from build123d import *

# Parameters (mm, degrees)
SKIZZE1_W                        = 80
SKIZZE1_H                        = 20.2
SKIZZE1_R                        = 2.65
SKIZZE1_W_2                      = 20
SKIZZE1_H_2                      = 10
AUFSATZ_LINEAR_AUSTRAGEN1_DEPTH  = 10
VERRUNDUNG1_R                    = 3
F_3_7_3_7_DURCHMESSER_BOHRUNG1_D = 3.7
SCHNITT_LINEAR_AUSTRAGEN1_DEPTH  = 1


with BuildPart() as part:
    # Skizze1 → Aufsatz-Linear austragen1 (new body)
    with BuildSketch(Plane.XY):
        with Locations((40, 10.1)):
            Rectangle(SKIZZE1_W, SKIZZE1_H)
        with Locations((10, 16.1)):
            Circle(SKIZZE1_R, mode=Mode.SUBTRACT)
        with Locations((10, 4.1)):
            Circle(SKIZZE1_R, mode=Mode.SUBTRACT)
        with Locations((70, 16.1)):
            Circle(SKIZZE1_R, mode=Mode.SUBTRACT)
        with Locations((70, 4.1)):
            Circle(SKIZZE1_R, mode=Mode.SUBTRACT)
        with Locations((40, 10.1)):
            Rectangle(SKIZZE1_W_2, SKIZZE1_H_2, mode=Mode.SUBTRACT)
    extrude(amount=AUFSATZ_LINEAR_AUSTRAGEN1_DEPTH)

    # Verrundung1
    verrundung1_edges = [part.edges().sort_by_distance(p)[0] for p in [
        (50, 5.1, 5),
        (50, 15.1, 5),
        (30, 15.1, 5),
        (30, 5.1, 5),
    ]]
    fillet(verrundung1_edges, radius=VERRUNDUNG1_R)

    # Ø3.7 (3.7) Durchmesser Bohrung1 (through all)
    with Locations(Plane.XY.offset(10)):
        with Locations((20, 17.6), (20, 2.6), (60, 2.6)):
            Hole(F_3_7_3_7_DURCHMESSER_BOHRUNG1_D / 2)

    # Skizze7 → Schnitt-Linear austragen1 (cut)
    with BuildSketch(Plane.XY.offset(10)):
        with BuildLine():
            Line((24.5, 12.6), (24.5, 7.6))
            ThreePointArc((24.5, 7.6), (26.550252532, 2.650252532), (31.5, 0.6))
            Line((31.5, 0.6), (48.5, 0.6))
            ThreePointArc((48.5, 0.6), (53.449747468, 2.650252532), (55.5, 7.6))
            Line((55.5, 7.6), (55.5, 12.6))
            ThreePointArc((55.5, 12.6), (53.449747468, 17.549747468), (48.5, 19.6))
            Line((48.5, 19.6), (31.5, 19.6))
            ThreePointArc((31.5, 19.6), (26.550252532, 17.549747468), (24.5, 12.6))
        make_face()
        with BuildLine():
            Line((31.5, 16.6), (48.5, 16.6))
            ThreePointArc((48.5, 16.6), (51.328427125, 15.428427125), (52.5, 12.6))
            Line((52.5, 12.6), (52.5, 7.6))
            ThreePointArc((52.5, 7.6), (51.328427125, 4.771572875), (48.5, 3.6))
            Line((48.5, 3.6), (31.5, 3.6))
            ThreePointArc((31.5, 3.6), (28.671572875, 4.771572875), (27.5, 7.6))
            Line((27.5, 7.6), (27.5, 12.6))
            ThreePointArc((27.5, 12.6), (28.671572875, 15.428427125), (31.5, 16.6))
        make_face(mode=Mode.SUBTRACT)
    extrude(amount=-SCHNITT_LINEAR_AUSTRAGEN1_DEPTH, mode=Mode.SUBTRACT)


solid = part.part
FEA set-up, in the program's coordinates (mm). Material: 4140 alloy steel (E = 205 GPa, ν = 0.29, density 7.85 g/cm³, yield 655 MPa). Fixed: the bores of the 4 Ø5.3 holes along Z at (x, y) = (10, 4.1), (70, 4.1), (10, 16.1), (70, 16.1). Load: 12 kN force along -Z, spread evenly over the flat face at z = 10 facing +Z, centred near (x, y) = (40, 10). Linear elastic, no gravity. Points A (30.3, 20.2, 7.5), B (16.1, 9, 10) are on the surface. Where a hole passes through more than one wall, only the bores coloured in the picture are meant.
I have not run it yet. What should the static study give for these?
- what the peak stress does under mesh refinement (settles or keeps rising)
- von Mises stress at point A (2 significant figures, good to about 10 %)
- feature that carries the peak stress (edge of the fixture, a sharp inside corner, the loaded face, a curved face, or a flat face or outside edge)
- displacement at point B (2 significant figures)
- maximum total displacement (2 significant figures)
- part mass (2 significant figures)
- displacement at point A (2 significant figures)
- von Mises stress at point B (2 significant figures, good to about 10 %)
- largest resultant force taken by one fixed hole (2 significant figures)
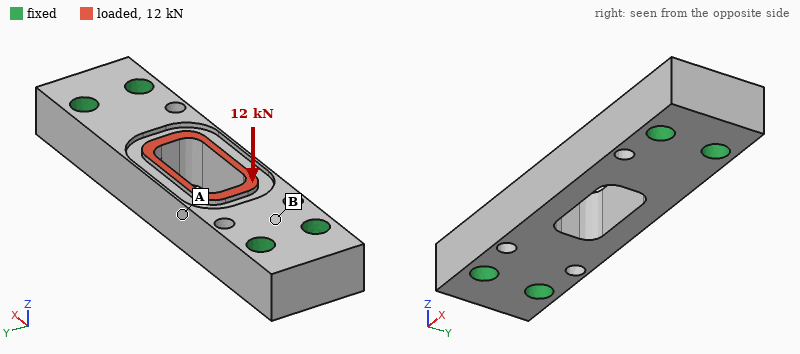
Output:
keeps rising
61 MPa
edge of the fixture
8.2 µm
53 µm
100 g
37 µm
180 MPa
3.0 kN
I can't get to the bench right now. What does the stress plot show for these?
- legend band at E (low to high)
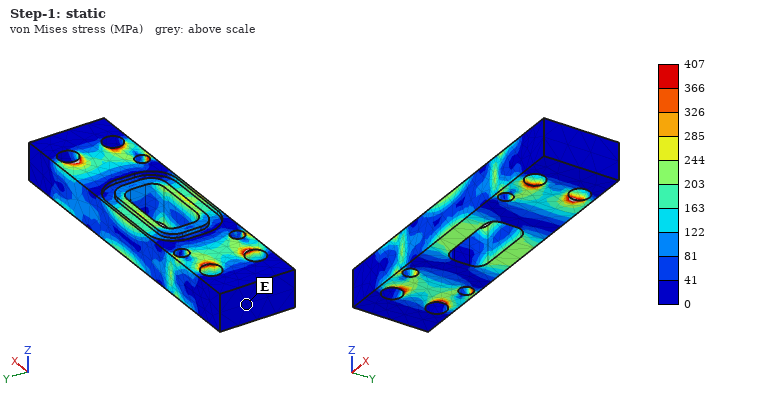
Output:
0 to 41 MPa
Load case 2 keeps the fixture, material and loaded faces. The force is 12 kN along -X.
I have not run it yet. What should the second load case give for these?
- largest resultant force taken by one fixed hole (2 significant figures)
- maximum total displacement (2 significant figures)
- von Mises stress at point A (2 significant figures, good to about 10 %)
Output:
3.4 kN
10 µm
26 MPa
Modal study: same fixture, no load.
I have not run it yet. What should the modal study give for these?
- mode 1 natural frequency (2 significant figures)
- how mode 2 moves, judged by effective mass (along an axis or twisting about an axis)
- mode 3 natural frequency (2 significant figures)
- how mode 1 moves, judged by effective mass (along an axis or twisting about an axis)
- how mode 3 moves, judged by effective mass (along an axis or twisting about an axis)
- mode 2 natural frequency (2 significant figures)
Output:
15 kHz
twisting about X
23 kHz
along Z
along Y
21 kHz
